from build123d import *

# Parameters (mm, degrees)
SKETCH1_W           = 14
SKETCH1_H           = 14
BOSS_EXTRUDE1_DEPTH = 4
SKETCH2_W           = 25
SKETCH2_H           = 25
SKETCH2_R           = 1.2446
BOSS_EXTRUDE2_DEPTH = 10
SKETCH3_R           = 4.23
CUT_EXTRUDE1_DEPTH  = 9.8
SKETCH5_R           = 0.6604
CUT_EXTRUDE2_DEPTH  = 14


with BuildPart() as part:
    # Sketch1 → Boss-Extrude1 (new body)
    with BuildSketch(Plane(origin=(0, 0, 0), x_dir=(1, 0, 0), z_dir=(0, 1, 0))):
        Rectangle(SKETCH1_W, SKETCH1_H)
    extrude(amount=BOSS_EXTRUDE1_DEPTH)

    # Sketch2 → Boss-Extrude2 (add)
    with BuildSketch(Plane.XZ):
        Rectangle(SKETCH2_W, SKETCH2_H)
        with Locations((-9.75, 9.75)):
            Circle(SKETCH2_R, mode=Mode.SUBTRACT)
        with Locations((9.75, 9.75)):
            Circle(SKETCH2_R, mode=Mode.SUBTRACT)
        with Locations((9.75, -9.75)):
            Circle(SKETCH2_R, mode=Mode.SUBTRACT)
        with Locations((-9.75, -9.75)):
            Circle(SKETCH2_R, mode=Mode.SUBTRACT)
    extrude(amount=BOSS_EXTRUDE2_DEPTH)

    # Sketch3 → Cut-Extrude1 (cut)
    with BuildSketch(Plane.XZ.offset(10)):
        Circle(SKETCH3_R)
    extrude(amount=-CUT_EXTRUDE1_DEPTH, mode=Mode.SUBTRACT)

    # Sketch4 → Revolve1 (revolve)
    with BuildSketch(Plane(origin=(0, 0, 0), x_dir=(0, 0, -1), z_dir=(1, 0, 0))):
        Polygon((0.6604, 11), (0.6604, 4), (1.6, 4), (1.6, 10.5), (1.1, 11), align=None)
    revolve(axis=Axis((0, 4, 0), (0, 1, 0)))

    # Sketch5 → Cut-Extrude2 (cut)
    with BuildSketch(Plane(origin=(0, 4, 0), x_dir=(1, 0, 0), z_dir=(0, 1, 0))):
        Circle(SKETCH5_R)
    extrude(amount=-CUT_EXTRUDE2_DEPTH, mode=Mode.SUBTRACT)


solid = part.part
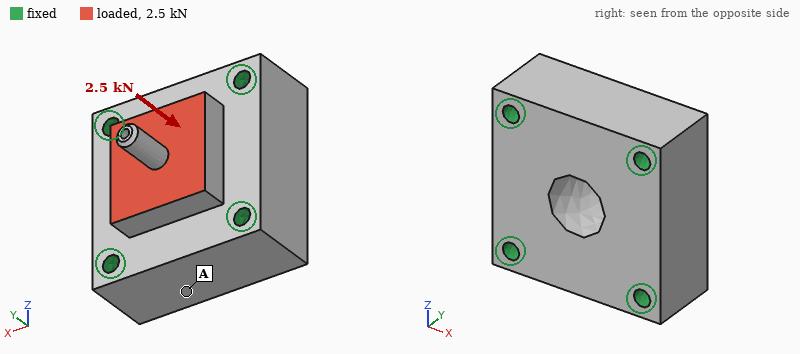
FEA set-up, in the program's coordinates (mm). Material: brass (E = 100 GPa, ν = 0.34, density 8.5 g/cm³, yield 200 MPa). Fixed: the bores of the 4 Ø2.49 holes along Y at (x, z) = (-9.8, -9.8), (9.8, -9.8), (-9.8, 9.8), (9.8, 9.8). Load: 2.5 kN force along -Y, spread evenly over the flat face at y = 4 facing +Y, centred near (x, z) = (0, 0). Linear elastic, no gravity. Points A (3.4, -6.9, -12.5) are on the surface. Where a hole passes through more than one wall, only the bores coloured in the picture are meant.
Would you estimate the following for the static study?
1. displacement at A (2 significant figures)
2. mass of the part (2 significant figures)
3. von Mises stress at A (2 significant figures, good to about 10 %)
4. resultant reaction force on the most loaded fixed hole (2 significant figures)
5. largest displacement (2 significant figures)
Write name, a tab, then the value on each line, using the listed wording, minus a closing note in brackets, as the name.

displacement at A	0.87 µm
mass of the part	54 g
von Mises stress at A	5.4 MPa
resultant reaction force on the most loaded fixed hole	660 N
largest displacement	2.8 µm
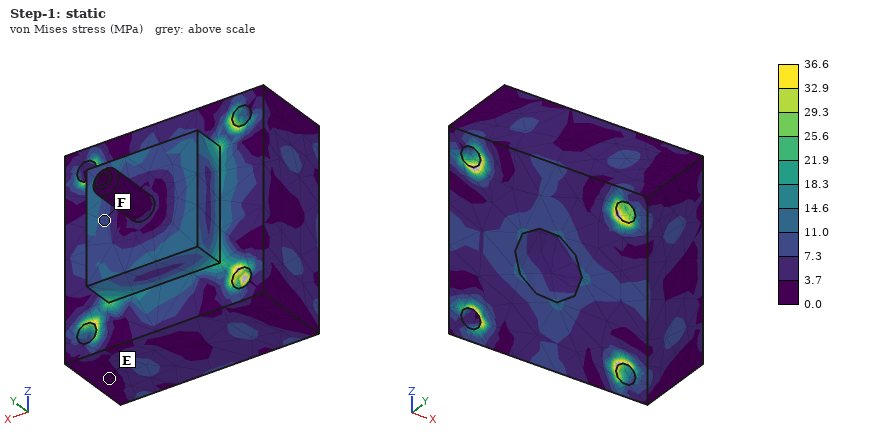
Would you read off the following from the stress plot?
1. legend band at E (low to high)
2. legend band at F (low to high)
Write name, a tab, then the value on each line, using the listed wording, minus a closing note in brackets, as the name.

legend band at E	0.0 to 3.7 MPa
legend band at F	7.3 to 11.0 MPa
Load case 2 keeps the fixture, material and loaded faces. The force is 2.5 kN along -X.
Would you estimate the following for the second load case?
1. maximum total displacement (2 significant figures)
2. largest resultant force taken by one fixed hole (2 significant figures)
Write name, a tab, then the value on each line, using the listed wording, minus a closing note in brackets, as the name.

maximum total displacement	5.9 µm
largest resultant force taken by one fixed hole	880 N
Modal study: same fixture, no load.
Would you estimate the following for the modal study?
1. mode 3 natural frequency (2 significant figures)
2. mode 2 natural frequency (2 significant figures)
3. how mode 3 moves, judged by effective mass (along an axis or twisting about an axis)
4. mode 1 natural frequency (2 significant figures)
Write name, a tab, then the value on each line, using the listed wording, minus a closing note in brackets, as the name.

mode 3 natural frequency	34 kHz
mode 2 natural frequency	26 kHz
how mode 3 moves, judged by effective mass	along Y
mode 1 natural frequency	26 kHz
